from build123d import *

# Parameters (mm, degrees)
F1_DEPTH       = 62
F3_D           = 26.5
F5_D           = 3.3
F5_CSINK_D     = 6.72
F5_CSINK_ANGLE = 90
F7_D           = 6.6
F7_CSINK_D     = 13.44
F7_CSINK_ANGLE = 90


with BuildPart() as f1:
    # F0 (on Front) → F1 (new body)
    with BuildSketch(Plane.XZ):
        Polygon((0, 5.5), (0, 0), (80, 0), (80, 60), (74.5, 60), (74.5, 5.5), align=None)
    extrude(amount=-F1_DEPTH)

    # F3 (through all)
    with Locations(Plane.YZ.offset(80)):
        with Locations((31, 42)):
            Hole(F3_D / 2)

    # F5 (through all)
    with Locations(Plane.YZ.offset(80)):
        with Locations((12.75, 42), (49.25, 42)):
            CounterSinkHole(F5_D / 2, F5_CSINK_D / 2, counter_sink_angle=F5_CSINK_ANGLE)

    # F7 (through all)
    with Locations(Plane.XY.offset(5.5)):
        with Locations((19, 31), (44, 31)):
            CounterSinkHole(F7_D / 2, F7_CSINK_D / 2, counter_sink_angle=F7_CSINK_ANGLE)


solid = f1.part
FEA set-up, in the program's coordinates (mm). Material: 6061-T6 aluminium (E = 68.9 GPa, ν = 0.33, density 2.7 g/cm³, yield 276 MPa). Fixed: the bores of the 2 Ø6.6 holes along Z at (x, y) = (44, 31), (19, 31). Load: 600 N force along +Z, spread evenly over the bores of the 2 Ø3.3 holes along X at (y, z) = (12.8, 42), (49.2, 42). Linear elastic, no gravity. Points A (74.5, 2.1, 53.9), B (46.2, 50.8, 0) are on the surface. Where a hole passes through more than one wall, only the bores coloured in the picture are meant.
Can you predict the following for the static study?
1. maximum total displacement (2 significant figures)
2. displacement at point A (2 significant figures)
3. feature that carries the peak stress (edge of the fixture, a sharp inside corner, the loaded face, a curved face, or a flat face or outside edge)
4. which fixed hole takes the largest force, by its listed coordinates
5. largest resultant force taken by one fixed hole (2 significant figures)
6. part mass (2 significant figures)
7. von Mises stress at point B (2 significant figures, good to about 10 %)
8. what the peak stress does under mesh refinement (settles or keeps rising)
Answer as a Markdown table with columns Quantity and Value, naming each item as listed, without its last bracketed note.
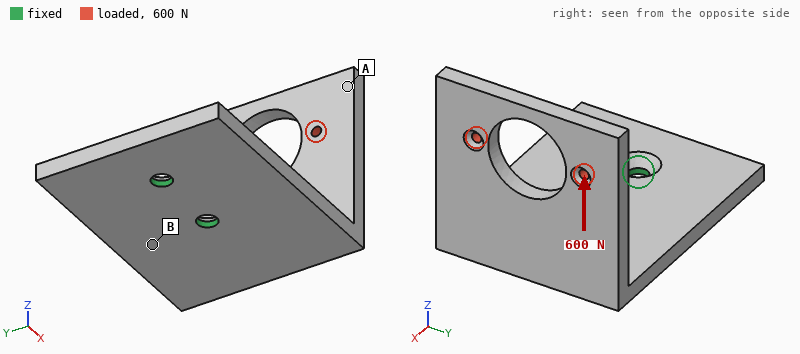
| Quantity | Value |
|---|---|
| maximum total displacement | 0.47 mm |
| displacement at point A | 0.42 mm |
| feature that carries the peak stress | edge of the fixture |
| which fixed hole takes the largest force, by its listed coordinates | (44, 31) |
| largest resultant force taken by one fixed hole | 1.4 kN |
| part mass | 110 g |
| von Mises stress at point B | 38 MPa |
| what the peak stress does under mesh refinement | keeps rising |
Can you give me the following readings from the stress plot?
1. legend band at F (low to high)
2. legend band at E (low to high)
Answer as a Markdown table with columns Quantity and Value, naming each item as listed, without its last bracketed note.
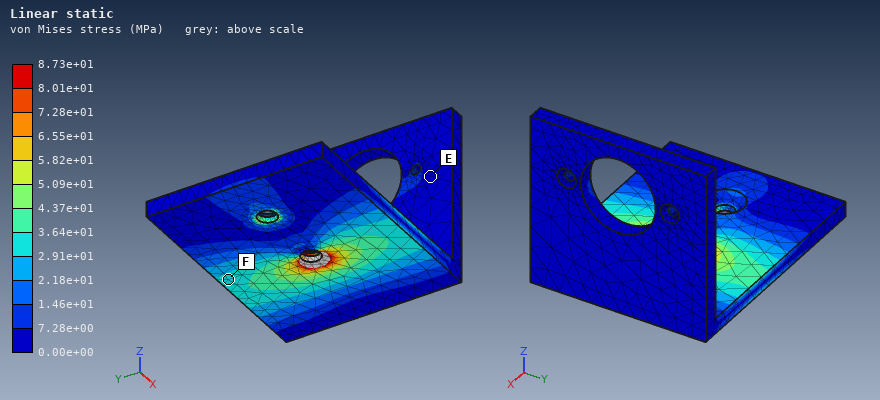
| Quantity | Value |
|---|---|
| legend band at F | 2.91e+01 to 3.64e+01 MPa |
| legend band at E | 0.00e+00 to 7.28e+00 MPa |
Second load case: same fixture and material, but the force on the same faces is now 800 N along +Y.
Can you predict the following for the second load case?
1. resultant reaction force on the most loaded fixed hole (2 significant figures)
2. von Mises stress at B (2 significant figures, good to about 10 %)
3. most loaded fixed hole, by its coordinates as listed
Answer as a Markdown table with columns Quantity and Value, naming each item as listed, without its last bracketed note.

| Quantity | Value |
|---|---|
| resultant reaction force on the most loaded fixed hole | 1.5 kN |
| von Mises stress at B | 54 MPa |
| most loaded fixed hole, by its coordinates as listed | (44, 31) |
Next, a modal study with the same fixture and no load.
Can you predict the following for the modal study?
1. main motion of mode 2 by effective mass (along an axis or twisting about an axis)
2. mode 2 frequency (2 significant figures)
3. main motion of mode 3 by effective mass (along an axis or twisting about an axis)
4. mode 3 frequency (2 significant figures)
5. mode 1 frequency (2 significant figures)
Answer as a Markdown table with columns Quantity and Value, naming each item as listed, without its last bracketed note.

| Quantity | Value |
|---|---|
| main motion of mode 2 by effective mass | along Y |
| mode 2 frequency | 820 Hz |
| main motion of mode 3 by effective mass | along Z |
| mode 3 frequency | 1900 Hz |
| mode 1 frequency | 710 Hz |
